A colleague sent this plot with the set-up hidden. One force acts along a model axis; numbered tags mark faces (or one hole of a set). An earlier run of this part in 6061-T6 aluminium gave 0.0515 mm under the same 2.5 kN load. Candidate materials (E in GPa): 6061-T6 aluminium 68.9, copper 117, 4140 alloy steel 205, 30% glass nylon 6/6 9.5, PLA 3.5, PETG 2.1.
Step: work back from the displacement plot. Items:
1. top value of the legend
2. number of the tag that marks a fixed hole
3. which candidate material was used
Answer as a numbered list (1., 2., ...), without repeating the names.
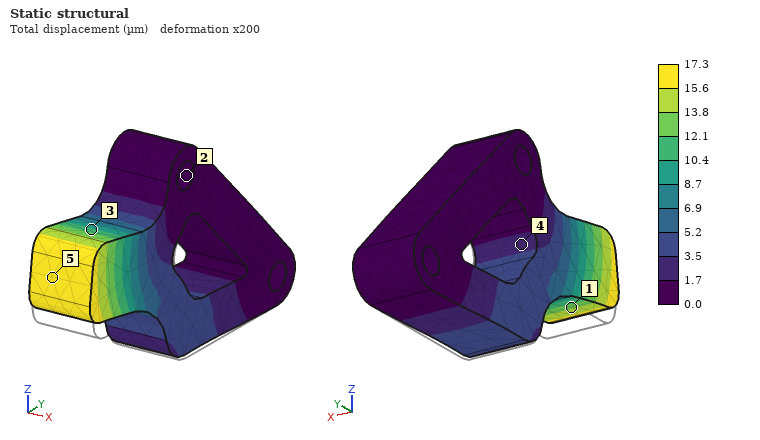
1. 17.3 µm
2. 2
3. 4140 alloy steel
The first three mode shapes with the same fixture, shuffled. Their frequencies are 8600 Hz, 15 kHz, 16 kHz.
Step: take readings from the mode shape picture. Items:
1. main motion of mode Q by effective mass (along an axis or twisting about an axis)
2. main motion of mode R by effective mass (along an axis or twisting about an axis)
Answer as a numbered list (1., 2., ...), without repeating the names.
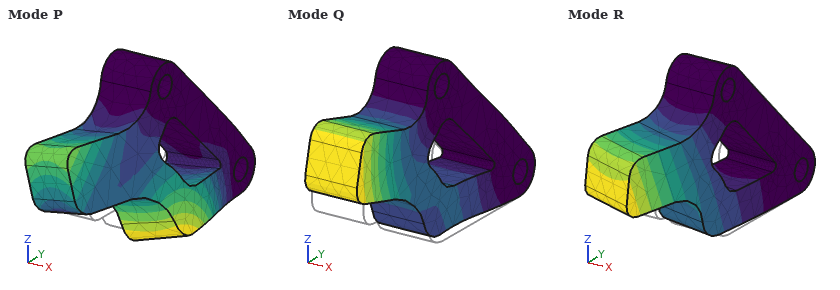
1. along Z
2. along X
